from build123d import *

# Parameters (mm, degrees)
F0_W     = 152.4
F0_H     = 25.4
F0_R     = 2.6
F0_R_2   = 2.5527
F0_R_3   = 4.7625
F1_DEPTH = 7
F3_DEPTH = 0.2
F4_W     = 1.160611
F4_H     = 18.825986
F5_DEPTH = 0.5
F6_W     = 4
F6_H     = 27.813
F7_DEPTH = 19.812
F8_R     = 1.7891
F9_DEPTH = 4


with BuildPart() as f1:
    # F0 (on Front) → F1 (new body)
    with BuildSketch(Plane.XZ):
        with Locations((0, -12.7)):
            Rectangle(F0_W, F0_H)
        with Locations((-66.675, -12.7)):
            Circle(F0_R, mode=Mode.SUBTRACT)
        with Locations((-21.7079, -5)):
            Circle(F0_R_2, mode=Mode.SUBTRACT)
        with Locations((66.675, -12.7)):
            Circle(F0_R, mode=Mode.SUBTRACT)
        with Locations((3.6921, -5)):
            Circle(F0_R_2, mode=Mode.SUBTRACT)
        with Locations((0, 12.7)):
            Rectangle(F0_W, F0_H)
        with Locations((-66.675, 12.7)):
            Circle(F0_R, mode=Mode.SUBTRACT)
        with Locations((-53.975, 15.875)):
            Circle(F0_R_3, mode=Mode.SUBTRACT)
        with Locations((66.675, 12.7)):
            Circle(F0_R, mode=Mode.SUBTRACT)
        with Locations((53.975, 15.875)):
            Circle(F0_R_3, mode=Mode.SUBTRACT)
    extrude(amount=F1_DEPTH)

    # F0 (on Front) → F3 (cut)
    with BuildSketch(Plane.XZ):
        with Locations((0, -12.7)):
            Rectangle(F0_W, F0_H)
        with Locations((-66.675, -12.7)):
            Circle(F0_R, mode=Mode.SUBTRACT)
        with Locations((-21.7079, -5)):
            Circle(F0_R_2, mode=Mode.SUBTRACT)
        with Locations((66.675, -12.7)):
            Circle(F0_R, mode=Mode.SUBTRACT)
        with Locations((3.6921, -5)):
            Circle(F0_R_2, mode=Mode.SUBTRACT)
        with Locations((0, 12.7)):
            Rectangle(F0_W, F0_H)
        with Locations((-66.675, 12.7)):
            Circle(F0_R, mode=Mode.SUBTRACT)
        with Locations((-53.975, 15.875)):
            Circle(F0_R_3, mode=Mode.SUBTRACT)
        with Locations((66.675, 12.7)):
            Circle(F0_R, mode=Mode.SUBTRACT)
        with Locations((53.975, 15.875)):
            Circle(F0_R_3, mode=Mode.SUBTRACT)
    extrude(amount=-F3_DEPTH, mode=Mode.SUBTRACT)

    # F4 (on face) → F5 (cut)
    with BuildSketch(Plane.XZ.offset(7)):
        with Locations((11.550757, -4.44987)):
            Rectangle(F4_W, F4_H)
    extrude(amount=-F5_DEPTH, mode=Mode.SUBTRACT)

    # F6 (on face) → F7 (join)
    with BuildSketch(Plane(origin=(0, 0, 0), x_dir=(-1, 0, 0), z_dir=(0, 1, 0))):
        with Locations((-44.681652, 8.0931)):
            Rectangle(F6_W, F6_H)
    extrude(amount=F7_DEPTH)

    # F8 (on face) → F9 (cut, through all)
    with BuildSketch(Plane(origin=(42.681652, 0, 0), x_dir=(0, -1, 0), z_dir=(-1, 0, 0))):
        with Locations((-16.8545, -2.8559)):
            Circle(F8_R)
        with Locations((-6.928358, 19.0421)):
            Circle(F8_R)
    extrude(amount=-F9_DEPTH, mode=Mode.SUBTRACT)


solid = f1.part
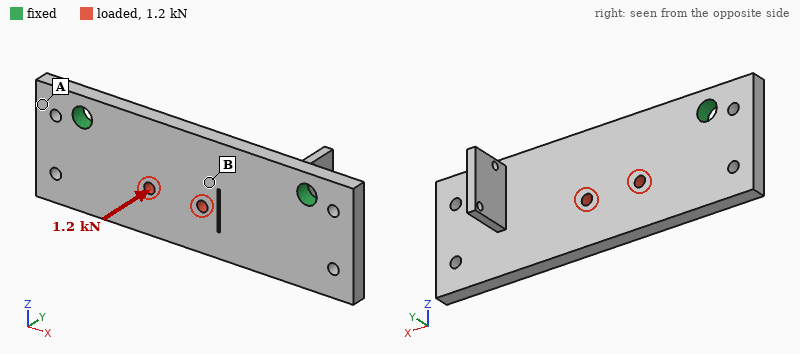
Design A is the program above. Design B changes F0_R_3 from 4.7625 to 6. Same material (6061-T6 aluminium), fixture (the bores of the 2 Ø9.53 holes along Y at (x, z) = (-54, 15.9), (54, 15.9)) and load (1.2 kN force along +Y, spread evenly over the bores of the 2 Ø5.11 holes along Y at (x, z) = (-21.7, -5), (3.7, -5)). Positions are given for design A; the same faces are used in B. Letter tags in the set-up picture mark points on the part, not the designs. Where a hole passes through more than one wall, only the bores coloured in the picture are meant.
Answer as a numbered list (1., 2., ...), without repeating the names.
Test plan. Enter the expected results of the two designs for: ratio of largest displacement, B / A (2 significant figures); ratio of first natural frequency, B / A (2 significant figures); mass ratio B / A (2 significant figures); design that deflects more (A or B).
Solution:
1. 0.89
2. 1.1
3. 0.99
4. A
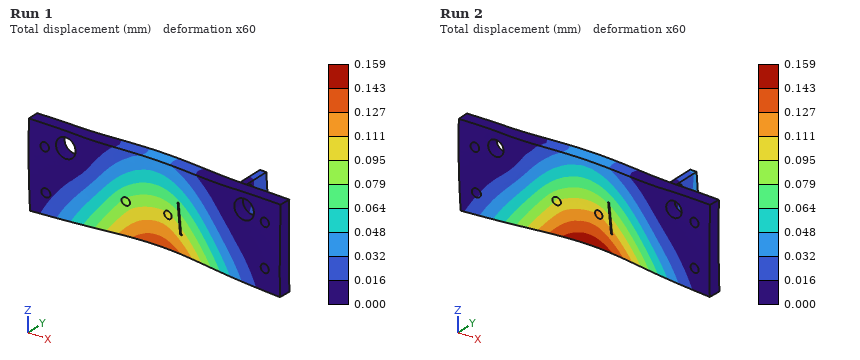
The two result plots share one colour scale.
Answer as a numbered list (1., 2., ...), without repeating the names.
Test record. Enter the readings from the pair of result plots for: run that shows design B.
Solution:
1. Run 1
